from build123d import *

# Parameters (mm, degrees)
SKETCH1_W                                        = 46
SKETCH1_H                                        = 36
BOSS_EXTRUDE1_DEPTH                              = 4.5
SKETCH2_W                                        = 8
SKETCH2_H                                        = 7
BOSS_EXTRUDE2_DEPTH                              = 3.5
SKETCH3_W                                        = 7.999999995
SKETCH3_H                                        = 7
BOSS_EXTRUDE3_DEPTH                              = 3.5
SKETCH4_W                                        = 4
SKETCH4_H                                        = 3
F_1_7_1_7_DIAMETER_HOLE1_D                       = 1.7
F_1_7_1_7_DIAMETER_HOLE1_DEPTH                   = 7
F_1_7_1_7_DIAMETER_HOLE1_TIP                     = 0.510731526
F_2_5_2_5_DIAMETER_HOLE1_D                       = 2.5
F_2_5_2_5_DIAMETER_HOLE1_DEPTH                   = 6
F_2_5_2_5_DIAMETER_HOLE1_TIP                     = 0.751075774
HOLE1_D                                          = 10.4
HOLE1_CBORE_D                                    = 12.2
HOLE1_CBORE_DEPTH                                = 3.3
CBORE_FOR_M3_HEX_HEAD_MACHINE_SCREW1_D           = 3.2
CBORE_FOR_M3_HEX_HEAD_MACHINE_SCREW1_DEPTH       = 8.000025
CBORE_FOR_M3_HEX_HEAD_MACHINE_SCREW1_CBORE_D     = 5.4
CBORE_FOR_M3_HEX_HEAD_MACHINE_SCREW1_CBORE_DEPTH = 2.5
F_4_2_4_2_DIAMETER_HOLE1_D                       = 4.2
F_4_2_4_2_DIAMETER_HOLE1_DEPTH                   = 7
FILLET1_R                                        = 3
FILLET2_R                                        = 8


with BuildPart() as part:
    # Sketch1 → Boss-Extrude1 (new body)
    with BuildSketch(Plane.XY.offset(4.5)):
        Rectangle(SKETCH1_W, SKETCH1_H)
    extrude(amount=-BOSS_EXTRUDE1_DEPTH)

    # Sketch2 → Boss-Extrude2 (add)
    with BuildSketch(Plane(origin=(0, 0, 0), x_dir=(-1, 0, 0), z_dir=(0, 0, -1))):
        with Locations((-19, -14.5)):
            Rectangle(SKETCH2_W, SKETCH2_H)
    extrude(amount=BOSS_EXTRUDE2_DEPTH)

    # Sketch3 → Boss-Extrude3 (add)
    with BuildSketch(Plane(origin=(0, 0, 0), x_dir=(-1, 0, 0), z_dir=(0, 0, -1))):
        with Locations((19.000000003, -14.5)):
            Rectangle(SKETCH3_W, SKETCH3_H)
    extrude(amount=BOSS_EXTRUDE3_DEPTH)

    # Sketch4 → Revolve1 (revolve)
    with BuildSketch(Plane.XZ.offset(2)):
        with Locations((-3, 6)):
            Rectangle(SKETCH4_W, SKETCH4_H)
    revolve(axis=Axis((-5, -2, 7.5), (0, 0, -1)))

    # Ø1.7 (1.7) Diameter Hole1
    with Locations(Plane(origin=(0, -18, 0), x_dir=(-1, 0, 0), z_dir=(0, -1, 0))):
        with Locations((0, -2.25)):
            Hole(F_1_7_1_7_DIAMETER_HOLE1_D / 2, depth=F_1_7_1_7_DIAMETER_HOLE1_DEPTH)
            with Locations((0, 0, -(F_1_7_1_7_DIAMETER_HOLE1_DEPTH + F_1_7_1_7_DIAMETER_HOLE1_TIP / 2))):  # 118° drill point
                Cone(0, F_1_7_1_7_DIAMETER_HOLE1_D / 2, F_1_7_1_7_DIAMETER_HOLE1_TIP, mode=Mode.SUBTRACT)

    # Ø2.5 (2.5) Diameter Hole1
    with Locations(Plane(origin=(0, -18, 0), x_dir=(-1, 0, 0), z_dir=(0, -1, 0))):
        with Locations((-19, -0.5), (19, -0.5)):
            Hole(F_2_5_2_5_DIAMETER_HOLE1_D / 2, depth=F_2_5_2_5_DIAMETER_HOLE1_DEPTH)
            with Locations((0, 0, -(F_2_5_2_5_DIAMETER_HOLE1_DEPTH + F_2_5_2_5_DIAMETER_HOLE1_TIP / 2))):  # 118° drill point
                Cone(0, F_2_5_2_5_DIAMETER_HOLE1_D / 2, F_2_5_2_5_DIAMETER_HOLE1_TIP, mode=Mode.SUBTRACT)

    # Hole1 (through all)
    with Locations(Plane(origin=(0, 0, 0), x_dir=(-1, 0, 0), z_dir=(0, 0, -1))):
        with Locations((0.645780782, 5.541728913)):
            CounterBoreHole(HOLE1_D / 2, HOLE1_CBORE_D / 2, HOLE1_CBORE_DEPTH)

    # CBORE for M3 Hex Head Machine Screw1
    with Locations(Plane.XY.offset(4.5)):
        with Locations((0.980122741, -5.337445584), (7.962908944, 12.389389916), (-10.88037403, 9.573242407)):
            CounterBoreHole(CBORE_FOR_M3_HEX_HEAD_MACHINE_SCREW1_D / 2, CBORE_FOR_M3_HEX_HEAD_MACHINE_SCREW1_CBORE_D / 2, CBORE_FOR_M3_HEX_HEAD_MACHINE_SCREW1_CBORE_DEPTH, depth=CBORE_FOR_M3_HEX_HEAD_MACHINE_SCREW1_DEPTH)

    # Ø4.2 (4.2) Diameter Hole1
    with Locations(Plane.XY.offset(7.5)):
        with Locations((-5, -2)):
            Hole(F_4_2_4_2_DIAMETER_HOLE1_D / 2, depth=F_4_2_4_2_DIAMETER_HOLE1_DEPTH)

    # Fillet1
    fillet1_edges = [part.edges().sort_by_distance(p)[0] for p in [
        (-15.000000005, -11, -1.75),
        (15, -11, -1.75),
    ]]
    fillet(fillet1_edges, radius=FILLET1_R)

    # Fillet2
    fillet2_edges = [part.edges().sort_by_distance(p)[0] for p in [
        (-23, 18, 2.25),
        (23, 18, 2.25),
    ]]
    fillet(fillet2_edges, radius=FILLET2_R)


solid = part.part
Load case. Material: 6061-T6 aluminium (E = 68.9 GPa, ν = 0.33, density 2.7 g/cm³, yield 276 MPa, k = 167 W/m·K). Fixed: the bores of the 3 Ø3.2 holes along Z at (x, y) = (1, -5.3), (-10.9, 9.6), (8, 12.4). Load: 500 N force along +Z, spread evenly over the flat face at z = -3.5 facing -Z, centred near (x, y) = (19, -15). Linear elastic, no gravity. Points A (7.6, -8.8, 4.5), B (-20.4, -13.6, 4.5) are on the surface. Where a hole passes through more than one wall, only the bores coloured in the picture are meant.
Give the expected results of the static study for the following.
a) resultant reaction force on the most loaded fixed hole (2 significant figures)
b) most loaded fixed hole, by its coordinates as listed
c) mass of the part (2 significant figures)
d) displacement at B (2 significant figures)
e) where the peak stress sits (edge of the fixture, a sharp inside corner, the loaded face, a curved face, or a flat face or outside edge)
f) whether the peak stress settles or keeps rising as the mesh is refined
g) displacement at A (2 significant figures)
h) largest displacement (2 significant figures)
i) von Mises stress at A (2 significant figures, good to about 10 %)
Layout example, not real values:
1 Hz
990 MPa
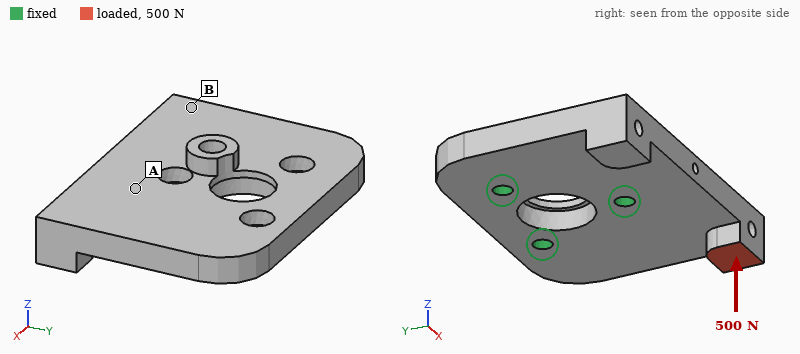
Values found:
810 N
(1, -5.3)
19 g
0.039 mm
edge of the fixture
keeps rising
0.050 mm
0.24 mm
49 MPa
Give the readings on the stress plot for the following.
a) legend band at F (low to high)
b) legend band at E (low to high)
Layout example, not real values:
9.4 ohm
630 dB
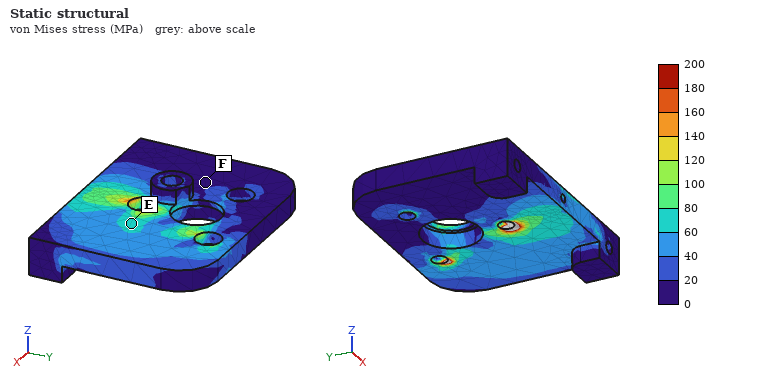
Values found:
0 to 20 MPa
60 to 80 MPa
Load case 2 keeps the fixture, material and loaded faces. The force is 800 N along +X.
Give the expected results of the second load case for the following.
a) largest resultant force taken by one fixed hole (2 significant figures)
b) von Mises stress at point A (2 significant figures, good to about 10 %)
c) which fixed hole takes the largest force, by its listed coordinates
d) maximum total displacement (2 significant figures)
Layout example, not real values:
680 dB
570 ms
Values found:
1.0 kN
33 MPa
(1, -5.3)
0.13 mm
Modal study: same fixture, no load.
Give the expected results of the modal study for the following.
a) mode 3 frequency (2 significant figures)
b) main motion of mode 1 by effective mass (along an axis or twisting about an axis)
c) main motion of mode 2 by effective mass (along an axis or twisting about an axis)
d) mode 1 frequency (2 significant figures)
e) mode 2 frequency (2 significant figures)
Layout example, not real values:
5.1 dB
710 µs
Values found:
13 kHz
twisting about Y
along Z
5000 Hz
6300 Hz
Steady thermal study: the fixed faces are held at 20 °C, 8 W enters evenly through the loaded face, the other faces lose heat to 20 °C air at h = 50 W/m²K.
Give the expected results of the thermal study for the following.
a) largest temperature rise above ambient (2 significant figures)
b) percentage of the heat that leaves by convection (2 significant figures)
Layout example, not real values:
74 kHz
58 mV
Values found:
16 K
7.4 %
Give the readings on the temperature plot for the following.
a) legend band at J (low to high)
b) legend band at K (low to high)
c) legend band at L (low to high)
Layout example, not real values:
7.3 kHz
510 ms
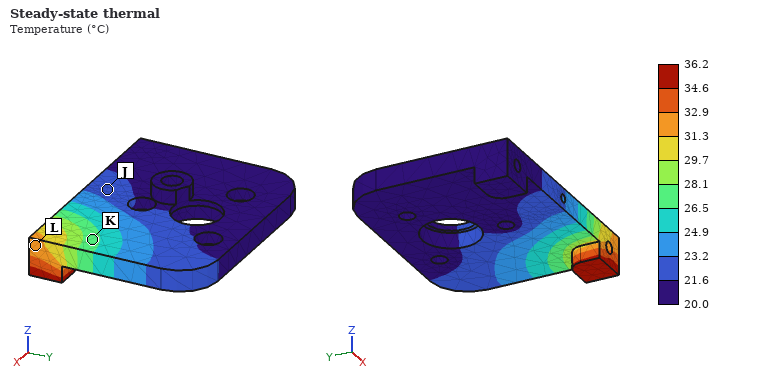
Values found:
21.6 to 23.2 °C
26.5 to 28.1 °C
31.3 to 32.9 °C
